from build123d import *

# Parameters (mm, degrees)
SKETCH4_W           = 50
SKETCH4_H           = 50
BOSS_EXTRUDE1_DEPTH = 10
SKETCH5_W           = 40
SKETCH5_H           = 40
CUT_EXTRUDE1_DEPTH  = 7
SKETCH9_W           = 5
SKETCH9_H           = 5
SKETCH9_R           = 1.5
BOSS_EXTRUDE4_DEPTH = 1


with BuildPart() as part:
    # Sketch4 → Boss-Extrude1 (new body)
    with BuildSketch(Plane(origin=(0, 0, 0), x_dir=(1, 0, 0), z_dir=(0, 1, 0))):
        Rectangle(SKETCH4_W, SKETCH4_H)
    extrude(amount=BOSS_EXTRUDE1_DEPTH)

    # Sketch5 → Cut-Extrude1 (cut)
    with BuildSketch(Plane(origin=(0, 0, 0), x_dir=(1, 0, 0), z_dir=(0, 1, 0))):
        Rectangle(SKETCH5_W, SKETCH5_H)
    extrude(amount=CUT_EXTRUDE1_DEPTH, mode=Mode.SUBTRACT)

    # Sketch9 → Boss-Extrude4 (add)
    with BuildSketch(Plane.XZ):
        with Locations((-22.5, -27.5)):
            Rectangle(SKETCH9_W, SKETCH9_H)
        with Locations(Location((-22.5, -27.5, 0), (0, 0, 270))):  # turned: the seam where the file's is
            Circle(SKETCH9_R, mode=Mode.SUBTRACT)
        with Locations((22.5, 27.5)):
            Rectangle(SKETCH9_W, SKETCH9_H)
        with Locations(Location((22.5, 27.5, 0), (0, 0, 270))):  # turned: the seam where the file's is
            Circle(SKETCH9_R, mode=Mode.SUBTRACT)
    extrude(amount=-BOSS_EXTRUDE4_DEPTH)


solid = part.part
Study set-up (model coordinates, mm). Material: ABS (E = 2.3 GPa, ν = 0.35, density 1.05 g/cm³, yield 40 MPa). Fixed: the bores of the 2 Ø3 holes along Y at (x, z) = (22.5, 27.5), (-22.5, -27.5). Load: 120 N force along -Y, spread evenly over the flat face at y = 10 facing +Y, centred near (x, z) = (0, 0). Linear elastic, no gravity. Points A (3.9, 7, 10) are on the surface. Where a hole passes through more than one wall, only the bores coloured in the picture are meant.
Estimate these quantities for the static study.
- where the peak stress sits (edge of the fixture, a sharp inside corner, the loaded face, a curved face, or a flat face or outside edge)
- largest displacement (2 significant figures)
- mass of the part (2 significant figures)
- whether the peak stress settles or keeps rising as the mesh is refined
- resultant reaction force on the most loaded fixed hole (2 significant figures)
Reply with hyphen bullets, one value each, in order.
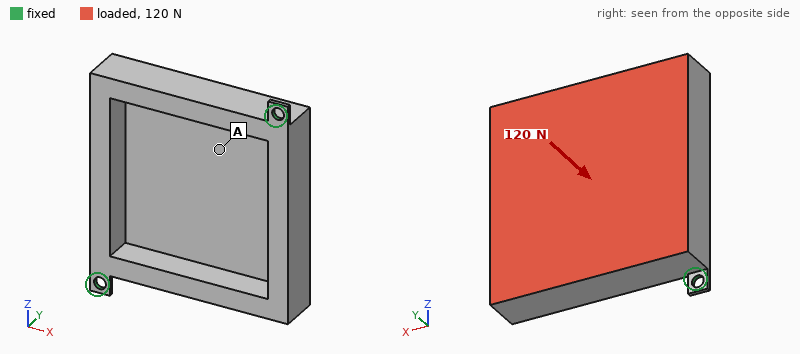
- edge of the fixture
- 0.38 mm
- 15 g
- keeps rising
- 120 N
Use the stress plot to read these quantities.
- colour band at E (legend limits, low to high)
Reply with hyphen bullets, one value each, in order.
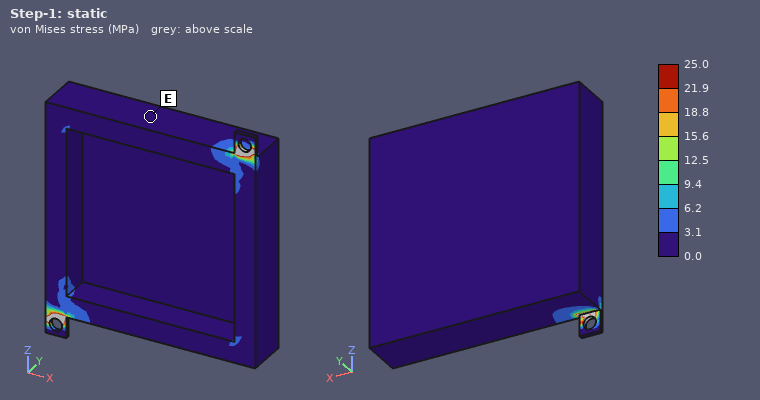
- 0.0 to 3.1 MPa
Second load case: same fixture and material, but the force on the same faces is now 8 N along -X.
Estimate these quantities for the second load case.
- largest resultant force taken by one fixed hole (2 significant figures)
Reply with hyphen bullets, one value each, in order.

- 4.0 N
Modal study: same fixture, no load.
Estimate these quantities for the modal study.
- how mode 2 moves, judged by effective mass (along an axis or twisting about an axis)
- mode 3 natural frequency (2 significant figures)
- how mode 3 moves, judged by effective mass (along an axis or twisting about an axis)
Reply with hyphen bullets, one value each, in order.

- along Y
- 1800 Hz
- along X
